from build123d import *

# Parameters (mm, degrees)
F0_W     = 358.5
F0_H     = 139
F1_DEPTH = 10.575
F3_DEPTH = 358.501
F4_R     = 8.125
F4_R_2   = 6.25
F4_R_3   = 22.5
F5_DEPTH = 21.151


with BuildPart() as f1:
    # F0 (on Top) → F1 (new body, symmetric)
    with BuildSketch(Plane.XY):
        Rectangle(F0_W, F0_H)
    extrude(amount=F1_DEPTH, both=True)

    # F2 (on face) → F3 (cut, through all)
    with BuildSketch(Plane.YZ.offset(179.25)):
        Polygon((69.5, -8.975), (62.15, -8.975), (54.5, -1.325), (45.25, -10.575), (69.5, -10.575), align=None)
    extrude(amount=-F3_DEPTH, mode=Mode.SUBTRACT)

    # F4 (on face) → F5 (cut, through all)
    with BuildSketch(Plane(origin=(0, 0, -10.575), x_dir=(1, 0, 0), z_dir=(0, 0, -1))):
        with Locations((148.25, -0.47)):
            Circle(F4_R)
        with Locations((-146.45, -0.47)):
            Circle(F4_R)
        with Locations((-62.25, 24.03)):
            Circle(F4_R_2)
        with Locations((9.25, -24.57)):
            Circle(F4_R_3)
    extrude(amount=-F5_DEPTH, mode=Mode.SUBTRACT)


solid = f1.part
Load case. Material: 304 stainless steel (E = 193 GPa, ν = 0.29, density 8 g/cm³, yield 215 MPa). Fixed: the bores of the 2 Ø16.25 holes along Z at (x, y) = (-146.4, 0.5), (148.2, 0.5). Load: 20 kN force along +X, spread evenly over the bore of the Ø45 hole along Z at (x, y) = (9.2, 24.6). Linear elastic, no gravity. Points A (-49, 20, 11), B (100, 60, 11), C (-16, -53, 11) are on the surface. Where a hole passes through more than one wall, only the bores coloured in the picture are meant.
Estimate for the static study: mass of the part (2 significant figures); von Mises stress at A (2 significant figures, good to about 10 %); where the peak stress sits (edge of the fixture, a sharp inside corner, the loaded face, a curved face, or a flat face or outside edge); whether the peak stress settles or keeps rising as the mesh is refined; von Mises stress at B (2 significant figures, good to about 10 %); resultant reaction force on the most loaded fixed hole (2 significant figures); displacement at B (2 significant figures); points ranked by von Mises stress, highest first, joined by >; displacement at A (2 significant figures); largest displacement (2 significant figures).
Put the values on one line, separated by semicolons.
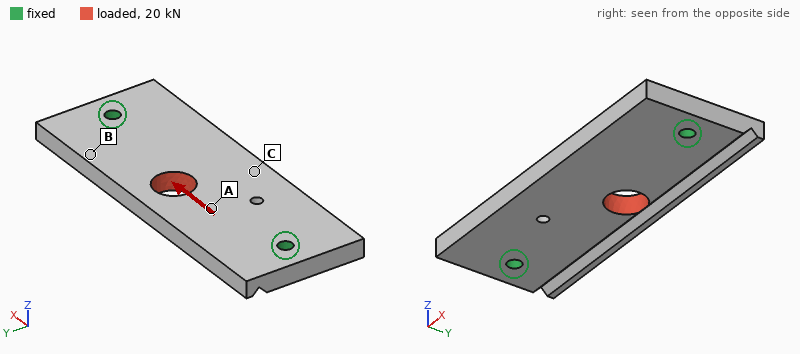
7.8 kg; 5.9 MPa; edge of the fixture; keeps rising; 3.3 MPa; 11 kN; 3.0 µm; A > B > C; 3.3 µm; 5.9 µm
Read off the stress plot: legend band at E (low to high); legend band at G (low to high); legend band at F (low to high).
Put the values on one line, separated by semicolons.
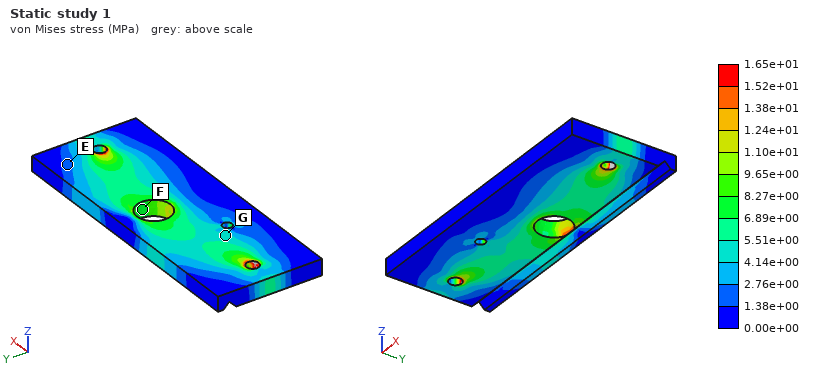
1.38e+00 to 2.76e+00 MPa; 4.14e+00 to 5.51e+00 MPa; 6.89e+00 to 8.27e+00 MPa
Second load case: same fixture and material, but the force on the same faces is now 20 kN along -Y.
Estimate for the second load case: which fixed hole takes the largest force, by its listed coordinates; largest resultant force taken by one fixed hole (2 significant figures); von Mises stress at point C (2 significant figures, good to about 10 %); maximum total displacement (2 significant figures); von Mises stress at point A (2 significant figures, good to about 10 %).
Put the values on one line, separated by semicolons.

(148.2, 0.5); 11 kN; 14 MPa; 24 µm; 7.7 MPa
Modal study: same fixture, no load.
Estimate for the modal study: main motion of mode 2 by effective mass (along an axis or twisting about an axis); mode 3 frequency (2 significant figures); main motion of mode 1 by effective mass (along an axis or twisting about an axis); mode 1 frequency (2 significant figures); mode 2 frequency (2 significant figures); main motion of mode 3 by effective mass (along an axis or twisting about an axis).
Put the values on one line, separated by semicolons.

twisting about X; 2600 Hz; along Z; 1000 Hz; 1400 Hz; twisting about Y
